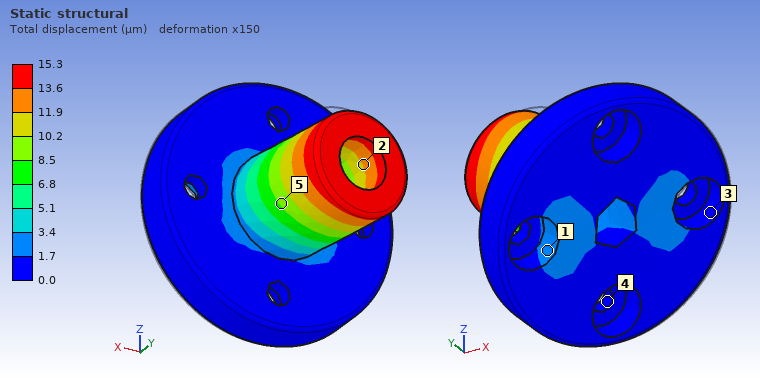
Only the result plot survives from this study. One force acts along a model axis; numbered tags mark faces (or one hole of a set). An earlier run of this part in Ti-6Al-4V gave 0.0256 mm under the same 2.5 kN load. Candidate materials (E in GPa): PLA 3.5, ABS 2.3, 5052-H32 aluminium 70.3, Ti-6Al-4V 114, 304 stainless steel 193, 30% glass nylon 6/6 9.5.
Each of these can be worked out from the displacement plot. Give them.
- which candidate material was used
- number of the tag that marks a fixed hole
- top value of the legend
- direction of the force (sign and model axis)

304 stainless steel
4
15.3 µm
-X
